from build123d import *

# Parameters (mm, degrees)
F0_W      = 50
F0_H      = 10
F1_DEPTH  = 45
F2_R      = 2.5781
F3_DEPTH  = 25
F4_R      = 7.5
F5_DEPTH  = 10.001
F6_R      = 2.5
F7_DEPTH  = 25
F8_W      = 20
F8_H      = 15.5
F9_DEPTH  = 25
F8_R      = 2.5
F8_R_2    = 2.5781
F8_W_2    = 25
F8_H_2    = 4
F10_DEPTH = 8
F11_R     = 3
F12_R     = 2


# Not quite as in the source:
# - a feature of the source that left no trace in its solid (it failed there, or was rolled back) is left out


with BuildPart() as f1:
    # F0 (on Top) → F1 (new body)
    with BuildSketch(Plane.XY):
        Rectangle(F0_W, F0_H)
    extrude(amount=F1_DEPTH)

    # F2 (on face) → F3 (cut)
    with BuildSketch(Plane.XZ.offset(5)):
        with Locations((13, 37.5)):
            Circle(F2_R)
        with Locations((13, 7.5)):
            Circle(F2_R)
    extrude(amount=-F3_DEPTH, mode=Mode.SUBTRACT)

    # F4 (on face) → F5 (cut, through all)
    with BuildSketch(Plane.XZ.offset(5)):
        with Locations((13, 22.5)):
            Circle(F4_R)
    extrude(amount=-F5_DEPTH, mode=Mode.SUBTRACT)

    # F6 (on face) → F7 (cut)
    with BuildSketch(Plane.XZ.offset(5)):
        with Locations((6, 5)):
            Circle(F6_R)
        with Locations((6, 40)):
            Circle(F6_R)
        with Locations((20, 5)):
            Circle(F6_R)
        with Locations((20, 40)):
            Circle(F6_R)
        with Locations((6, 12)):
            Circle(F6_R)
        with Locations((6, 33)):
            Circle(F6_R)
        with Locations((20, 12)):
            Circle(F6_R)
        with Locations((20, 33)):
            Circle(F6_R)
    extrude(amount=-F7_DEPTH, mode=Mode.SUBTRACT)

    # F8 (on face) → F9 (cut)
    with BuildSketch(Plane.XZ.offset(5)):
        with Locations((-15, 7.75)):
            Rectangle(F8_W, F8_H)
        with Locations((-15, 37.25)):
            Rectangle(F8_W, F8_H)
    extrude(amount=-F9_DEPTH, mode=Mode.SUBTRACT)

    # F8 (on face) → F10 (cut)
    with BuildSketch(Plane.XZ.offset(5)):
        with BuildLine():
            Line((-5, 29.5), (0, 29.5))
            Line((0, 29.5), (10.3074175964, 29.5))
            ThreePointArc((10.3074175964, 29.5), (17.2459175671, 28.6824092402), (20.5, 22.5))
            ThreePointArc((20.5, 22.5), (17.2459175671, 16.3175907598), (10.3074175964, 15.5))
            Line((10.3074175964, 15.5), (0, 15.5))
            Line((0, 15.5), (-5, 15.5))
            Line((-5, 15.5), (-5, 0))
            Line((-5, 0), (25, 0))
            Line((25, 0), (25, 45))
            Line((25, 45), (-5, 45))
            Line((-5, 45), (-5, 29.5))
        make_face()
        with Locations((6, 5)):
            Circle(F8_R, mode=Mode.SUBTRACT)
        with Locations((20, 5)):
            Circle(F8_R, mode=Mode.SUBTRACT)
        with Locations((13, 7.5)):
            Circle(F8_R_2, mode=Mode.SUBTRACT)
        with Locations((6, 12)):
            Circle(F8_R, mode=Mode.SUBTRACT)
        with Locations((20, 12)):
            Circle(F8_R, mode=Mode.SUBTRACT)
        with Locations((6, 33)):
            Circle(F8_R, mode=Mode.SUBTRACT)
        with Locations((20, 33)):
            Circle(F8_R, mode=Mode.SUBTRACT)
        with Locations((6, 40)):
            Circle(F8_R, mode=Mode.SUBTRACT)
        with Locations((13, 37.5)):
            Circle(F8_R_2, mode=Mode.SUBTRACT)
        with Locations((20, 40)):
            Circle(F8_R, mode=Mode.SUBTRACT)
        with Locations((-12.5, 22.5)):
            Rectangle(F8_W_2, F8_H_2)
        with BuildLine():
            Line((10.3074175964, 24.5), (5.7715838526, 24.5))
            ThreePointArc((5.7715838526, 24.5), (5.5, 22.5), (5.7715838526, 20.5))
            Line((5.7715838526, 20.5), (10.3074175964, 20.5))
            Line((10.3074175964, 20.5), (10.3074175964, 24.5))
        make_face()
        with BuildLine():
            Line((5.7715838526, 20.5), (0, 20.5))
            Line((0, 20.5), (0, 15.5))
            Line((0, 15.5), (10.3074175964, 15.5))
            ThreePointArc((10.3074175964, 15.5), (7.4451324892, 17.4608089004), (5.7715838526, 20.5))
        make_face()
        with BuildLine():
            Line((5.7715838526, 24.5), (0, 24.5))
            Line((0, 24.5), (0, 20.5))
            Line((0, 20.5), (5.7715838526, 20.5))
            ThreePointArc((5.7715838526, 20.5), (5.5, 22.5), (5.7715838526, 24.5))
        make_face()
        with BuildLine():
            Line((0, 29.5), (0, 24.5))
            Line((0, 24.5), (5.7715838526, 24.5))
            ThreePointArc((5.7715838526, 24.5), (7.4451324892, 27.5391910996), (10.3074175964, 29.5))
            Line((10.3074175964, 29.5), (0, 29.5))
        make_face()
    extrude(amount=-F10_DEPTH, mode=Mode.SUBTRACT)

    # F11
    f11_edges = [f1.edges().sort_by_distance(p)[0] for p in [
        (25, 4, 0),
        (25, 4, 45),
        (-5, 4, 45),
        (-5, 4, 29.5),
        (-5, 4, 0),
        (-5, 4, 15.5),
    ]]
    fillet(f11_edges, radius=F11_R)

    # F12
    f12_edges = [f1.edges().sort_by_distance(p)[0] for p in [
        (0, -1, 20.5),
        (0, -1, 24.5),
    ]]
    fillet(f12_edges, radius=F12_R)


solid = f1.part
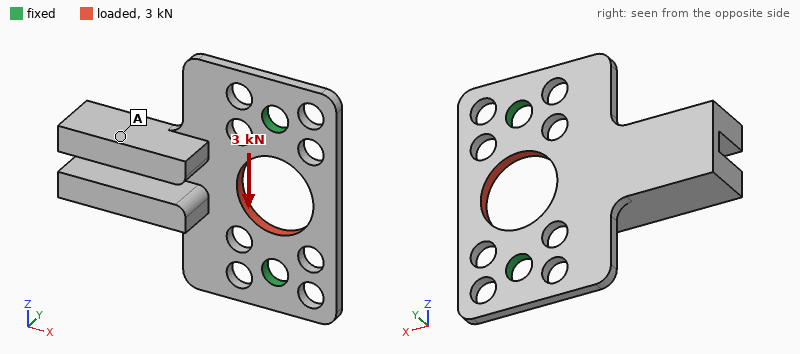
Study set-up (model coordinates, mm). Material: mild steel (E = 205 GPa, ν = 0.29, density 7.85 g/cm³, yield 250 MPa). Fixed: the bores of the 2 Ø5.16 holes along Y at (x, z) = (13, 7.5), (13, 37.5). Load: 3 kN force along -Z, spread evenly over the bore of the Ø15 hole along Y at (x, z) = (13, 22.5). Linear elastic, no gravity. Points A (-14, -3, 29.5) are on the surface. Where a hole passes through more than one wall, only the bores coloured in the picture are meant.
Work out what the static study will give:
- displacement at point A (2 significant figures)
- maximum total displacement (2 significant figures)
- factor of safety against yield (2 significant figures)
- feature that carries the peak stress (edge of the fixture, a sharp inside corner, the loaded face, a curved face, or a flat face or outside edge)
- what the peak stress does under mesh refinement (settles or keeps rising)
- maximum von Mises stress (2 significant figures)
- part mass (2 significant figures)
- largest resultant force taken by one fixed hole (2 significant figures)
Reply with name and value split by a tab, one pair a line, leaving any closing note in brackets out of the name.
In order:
displacement at point A	2.5 µm
maximum total displacement	7.4 µm
factor of safety against yield	1.2
feature that carries the peak stress	a curved face
what the peak stress does under mesh refinement	settles
maximum von Mises stress	220 MPa
part mass	35 g
largest resultant force taken by one fixed hole	1.5 kN
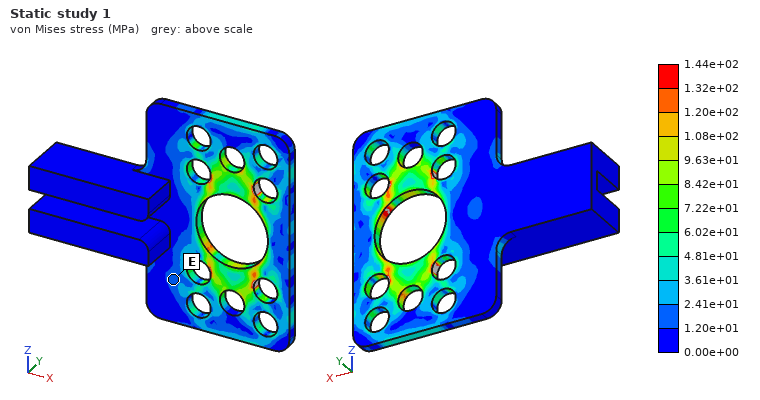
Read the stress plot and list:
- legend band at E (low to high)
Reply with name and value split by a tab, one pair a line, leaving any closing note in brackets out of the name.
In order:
legend band at E	1.20e+01 to 2.41e+01 MPa
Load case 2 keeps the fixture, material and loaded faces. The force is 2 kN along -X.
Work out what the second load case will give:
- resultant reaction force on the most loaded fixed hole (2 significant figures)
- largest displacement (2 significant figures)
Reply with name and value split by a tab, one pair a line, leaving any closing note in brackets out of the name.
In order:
resultant reaction force on the most loaded fixed hole	1.0 kN
largest displacement	6.8 µm
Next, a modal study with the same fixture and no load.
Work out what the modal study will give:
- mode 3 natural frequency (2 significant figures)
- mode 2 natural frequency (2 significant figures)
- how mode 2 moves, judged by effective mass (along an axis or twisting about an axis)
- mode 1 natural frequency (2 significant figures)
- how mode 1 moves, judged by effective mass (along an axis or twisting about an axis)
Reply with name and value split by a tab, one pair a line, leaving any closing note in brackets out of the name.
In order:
mode 3 natural frequency	6300 Hz
mode 2 natural frequency	4400 Hz
how mode 2 moves, judged by effective mass	along Z
mode 1 natural frequency	770 Hz
how mode 1 moves, judged by effective mass	along Y
